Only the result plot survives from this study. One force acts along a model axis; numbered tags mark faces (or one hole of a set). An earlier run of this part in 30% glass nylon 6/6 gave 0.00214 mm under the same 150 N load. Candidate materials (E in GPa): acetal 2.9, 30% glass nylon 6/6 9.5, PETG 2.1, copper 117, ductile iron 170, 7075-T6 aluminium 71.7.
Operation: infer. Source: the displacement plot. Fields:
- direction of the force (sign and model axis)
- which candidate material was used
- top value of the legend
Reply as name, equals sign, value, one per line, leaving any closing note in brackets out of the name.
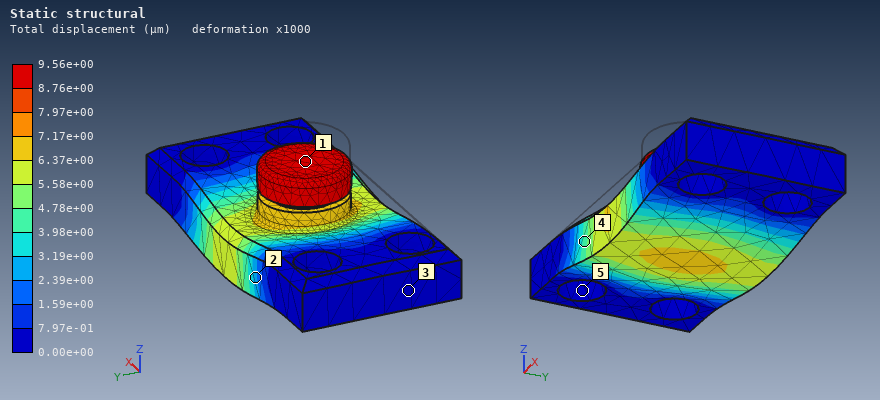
direction of the force = -Z
which candidate material was used = PETG
top value of the legend = 9.56e+00 µm
